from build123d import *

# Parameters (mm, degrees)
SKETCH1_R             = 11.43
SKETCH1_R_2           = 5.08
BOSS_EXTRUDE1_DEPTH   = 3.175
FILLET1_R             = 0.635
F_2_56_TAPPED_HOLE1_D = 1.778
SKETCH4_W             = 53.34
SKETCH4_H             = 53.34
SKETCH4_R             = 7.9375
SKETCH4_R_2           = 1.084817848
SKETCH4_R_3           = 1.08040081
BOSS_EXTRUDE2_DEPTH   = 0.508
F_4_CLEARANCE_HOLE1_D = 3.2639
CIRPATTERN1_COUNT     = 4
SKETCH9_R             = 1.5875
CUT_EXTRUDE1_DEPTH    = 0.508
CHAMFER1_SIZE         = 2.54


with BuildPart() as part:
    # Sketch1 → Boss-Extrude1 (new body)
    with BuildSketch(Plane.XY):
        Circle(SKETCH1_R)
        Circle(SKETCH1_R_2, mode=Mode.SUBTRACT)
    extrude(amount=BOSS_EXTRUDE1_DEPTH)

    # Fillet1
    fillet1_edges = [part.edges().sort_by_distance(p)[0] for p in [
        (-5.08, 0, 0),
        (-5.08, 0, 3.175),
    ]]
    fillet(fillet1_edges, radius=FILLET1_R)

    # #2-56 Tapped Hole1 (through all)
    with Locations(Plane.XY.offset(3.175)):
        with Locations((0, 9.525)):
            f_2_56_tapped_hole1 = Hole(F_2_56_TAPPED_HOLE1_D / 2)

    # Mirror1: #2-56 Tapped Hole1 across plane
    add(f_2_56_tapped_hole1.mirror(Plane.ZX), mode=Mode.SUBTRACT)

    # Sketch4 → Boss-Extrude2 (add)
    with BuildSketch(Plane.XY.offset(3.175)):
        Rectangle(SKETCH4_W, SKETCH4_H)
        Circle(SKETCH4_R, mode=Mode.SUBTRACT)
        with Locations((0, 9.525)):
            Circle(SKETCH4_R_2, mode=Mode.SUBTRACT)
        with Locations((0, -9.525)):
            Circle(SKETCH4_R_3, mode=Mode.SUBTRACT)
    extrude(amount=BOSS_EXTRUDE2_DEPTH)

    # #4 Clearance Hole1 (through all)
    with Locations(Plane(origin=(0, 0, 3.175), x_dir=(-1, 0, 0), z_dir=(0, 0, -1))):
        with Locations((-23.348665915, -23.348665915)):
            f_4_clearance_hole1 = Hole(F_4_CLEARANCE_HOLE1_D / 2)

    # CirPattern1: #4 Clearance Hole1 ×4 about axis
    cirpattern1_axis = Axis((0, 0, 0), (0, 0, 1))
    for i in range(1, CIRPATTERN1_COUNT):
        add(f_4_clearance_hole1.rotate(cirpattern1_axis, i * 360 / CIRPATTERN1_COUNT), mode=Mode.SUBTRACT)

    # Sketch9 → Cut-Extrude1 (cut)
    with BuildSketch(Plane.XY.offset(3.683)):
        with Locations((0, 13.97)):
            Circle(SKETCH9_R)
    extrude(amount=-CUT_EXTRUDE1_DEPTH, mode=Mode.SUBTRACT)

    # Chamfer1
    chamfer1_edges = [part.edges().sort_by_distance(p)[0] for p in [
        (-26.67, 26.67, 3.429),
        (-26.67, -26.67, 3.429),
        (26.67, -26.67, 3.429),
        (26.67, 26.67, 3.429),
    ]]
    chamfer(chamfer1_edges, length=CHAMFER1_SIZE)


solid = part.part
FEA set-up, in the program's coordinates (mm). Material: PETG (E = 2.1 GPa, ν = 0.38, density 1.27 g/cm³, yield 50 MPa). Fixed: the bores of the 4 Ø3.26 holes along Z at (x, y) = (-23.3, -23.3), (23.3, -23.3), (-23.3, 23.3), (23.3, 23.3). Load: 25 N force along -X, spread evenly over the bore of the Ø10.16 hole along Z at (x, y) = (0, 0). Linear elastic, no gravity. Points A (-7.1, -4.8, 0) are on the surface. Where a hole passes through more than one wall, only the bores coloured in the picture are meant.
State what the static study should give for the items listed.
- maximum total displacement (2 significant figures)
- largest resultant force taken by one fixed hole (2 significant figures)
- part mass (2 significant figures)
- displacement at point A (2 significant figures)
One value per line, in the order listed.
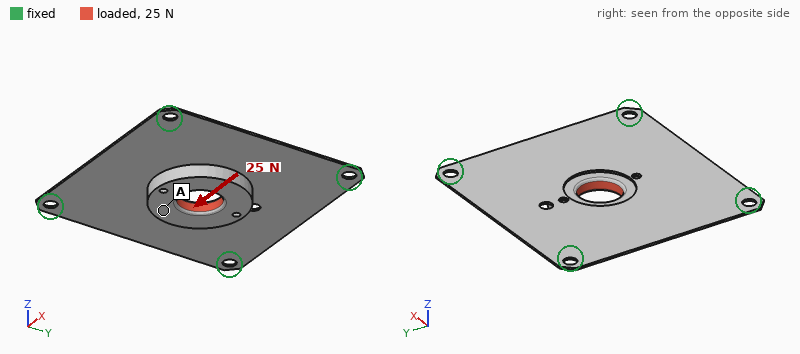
0.82 mm
7.2 N
3.0 g
0.46 mm
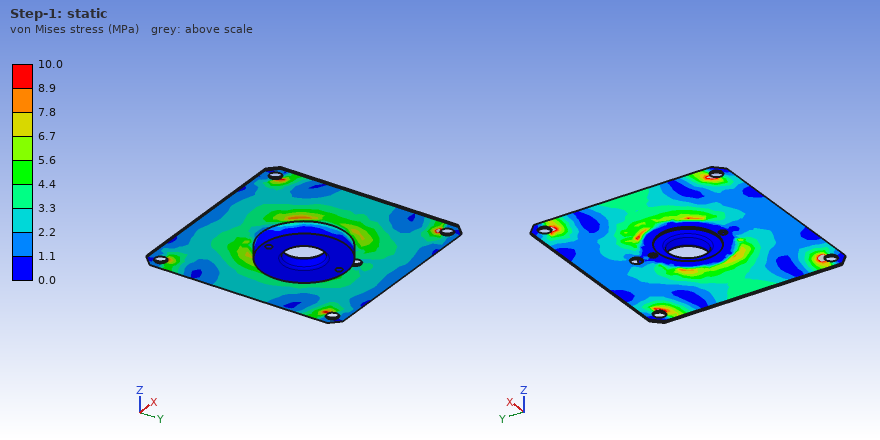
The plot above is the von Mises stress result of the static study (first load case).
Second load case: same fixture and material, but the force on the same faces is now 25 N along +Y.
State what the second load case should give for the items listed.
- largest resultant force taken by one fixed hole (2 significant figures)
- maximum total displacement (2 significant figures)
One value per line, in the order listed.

7.1 N
0.82 mm
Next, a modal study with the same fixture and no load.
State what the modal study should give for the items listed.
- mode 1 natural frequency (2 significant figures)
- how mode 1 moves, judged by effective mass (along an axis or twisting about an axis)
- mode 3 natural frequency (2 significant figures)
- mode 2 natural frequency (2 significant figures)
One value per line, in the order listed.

180 Hz
along Z
350 Hz
350 Hz
